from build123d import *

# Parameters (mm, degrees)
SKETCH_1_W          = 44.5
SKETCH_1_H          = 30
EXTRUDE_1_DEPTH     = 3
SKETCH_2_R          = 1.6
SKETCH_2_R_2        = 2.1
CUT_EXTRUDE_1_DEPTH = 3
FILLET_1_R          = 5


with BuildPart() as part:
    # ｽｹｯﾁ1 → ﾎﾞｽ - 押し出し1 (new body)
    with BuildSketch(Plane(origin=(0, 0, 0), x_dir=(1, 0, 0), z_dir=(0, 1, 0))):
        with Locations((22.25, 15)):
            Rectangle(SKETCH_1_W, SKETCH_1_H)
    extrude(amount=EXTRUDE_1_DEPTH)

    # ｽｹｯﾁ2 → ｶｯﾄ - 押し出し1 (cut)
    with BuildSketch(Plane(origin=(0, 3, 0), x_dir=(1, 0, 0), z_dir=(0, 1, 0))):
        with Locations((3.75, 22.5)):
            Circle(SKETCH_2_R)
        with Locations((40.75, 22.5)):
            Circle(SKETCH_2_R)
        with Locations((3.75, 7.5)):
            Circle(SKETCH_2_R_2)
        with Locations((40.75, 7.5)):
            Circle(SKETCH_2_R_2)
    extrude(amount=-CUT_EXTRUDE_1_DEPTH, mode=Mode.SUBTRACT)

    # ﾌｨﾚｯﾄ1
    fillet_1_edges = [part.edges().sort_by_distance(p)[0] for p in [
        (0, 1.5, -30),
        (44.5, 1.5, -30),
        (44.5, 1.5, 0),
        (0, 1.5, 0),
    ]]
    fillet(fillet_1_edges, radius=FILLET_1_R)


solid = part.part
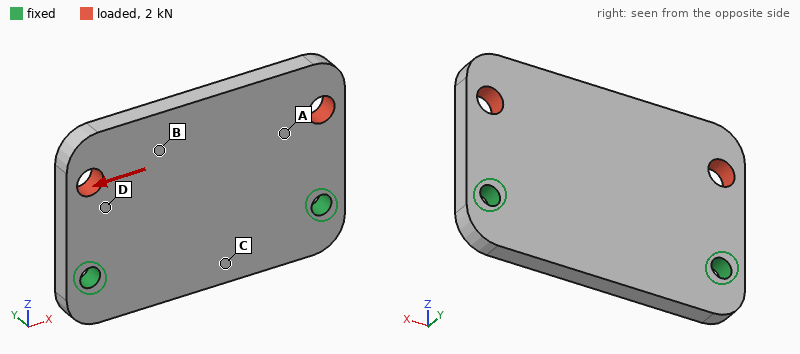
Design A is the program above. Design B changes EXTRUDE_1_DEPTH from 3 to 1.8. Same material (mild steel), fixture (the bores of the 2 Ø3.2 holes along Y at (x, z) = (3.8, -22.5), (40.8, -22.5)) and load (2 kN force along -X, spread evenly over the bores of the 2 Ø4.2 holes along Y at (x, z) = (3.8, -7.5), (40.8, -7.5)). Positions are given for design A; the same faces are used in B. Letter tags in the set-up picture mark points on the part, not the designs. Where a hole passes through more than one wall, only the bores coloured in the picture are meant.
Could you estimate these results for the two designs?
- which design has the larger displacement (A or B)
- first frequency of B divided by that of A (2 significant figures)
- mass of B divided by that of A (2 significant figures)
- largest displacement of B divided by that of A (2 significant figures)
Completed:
B
0.63
0.60
1.7
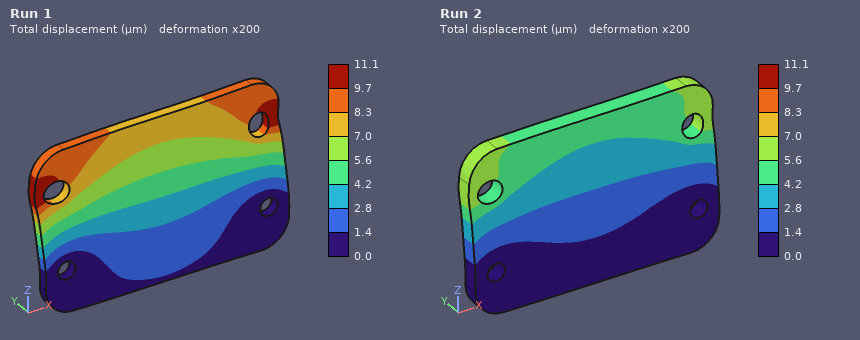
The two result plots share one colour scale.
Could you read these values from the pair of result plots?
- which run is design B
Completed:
Run 1
